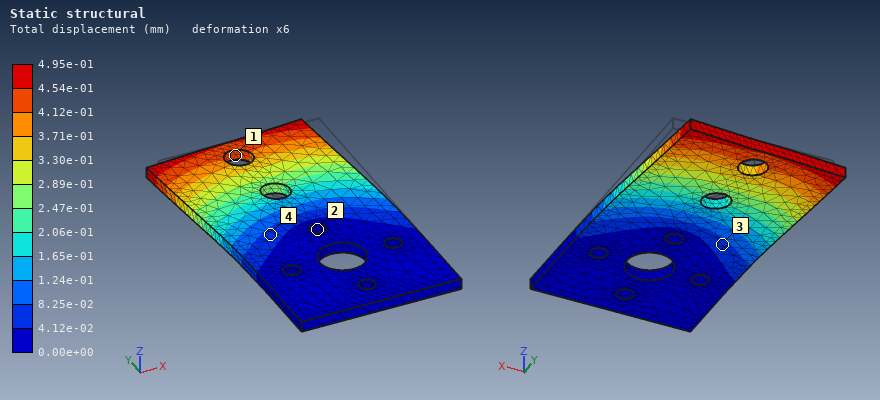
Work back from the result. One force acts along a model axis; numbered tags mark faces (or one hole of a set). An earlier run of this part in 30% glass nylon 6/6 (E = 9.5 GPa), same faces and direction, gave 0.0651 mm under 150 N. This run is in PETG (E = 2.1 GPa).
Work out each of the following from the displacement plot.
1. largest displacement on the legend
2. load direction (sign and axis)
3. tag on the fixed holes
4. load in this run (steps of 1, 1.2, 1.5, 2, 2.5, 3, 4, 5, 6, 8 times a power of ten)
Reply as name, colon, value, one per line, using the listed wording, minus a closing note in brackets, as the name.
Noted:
largest displacement on the legend: 4.95e-01 mm
load direction: -X
tag on the fixed holes: 2
load in this run: 250 N
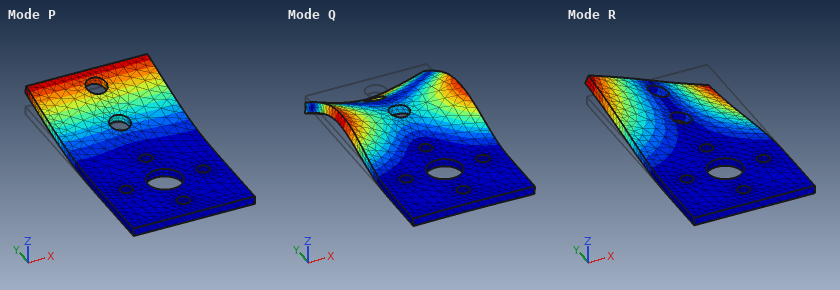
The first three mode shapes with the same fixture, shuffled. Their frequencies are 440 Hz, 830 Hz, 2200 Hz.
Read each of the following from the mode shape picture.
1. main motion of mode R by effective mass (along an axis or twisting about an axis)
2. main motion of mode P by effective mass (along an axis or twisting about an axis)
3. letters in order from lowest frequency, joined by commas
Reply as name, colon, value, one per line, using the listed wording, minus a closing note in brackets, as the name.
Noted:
main motion of mode R by effective mass: twisting about Y
main motion of mode P by effective mass: along Z
letters in order from lowest frequency, joined by commas: P, R, Q
